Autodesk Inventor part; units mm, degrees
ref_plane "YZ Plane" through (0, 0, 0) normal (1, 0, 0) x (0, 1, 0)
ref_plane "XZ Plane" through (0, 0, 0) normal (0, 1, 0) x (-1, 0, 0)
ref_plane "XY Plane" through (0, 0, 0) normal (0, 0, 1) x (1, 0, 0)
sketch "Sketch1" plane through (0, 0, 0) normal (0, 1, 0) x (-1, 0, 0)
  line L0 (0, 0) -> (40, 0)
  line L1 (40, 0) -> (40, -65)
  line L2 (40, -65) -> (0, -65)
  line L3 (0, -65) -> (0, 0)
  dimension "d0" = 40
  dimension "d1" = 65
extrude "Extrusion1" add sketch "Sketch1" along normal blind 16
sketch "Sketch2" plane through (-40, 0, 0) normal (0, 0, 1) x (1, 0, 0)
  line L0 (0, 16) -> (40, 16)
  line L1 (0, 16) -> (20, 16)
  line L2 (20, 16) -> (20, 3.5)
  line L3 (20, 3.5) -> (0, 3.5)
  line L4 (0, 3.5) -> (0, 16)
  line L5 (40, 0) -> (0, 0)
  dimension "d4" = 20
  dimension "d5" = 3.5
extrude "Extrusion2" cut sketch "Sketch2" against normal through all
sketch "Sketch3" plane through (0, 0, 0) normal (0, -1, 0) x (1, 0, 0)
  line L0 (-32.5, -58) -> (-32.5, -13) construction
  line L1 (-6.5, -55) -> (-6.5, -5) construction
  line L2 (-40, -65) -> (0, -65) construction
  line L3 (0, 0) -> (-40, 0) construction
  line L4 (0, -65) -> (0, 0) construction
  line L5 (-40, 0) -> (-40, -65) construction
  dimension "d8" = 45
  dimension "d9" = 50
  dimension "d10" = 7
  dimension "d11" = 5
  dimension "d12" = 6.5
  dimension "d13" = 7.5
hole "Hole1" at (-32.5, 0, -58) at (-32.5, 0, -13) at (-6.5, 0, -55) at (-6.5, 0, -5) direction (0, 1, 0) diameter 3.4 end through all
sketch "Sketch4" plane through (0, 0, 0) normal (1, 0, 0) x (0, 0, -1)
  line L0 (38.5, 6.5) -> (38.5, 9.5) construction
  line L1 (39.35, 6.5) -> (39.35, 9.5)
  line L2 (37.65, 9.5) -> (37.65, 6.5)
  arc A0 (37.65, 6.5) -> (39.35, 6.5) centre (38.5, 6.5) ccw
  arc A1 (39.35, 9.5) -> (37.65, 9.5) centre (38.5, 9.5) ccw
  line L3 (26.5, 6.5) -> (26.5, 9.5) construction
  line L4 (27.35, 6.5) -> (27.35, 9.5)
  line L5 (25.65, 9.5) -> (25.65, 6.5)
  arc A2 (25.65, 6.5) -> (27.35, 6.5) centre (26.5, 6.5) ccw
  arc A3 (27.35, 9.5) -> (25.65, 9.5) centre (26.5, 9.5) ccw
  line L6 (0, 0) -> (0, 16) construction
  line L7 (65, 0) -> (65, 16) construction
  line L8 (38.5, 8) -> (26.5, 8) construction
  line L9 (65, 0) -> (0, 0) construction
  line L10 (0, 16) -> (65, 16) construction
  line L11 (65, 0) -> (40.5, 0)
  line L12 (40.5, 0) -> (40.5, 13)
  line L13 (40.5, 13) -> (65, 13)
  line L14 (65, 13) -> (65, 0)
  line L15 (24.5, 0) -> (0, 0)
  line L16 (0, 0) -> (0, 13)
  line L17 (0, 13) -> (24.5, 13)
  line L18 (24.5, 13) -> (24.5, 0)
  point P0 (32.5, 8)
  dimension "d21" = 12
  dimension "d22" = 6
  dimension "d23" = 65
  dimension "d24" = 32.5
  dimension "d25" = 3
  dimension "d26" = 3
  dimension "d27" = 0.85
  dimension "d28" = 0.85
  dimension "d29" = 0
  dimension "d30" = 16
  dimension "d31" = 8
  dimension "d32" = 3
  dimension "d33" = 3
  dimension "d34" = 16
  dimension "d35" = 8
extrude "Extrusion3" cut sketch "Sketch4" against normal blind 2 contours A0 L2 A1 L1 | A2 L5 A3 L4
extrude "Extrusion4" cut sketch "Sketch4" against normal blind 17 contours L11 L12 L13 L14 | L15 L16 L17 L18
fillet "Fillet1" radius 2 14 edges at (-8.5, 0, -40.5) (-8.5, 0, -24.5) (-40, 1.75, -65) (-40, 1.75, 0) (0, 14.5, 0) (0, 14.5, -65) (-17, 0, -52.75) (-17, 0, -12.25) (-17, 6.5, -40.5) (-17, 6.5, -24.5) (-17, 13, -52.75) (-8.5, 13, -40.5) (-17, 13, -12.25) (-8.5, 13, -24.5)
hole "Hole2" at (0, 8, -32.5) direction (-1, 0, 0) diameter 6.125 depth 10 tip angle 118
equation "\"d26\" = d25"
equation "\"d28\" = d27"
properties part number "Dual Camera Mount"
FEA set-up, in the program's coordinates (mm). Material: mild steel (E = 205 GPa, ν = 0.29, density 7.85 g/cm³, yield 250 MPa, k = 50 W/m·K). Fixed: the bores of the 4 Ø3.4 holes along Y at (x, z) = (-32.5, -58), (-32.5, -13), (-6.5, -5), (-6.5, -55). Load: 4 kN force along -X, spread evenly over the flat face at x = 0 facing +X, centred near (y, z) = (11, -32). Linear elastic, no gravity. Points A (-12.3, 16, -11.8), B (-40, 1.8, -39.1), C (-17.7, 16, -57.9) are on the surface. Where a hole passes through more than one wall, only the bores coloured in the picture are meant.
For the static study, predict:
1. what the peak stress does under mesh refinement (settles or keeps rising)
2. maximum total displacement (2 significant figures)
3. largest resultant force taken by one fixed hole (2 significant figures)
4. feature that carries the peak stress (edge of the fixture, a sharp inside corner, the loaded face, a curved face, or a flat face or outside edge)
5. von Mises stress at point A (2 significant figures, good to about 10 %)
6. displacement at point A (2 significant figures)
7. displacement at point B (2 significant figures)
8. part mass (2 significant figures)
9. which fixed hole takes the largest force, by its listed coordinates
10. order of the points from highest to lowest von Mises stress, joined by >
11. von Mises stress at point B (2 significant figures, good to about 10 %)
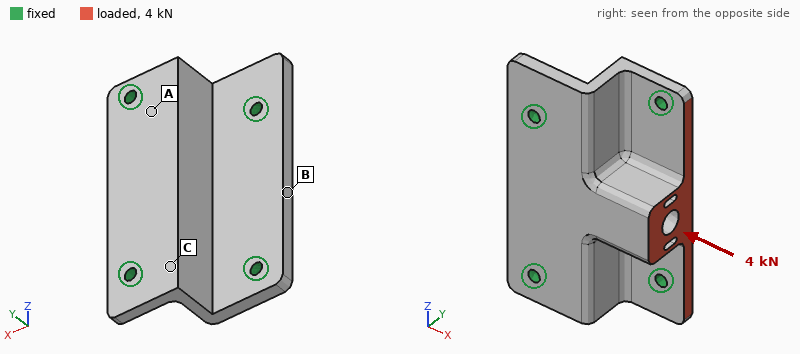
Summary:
keeps rising
9.6 µm
1.5 kN
edge of the fixture
34 MPa
3.4 µm
3.0 µm
110 g
(-6.5, -55)
A > B > C
18 MPa
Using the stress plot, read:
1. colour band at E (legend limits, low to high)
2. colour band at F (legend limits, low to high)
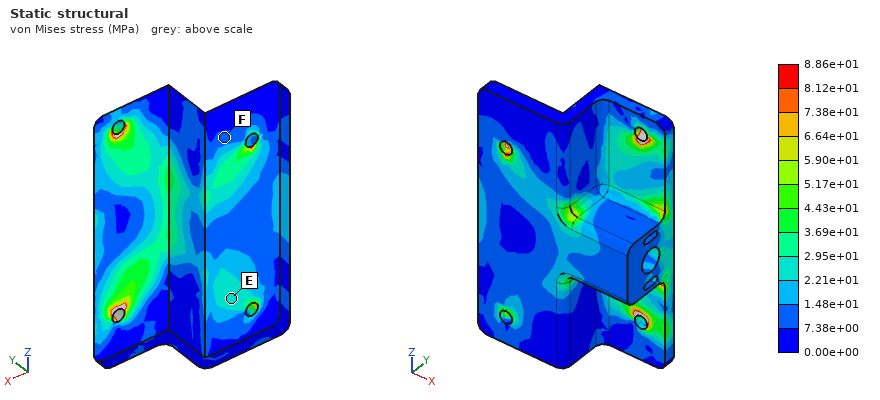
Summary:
2.21e+01 to 2.95e+01 MPa
7.38e+00 to 1.48e+01 MPa
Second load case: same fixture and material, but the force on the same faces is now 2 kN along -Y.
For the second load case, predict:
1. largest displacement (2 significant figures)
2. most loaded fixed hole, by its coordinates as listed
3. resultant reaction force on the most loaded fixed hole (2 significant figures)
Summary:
31 µm
(-6.5, -55)
1.2 kN
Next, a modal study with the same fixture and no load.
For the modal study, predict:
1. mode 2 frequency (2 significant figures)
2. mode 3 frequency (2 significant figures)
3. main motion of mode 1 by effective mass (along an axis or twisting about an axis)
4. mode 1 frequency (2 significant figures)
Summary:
11 kHz
14 kHz
along Y
6700 Hz
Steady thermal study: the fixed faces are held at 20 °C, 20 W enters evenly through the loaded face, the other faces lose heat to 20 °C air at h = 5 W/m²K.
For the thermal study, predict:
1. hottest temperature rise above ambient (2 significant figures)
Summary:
38 K
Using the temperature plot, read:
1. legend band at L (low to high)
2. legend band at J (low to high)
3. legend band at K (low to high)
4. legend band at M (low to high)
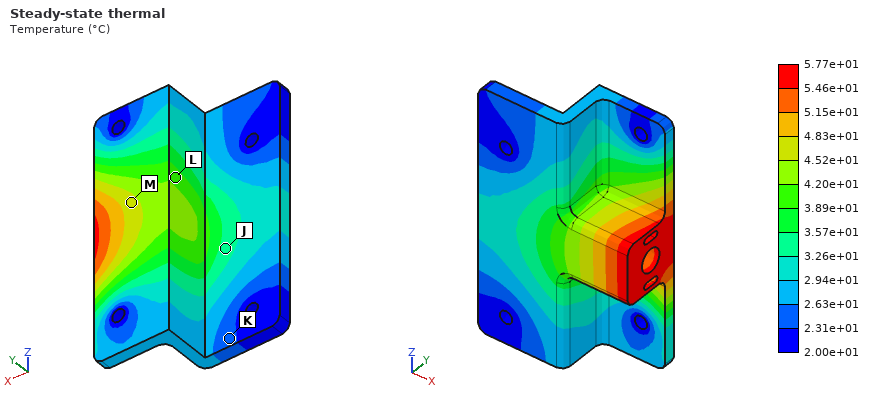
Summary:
3.89e+01 to 4.20e+01 °C
3.26e+01 to 3.57e+01 °C
2.31e+01 to 2.63e+01 °C
4.52e+01 to 4.83e+01 °C
